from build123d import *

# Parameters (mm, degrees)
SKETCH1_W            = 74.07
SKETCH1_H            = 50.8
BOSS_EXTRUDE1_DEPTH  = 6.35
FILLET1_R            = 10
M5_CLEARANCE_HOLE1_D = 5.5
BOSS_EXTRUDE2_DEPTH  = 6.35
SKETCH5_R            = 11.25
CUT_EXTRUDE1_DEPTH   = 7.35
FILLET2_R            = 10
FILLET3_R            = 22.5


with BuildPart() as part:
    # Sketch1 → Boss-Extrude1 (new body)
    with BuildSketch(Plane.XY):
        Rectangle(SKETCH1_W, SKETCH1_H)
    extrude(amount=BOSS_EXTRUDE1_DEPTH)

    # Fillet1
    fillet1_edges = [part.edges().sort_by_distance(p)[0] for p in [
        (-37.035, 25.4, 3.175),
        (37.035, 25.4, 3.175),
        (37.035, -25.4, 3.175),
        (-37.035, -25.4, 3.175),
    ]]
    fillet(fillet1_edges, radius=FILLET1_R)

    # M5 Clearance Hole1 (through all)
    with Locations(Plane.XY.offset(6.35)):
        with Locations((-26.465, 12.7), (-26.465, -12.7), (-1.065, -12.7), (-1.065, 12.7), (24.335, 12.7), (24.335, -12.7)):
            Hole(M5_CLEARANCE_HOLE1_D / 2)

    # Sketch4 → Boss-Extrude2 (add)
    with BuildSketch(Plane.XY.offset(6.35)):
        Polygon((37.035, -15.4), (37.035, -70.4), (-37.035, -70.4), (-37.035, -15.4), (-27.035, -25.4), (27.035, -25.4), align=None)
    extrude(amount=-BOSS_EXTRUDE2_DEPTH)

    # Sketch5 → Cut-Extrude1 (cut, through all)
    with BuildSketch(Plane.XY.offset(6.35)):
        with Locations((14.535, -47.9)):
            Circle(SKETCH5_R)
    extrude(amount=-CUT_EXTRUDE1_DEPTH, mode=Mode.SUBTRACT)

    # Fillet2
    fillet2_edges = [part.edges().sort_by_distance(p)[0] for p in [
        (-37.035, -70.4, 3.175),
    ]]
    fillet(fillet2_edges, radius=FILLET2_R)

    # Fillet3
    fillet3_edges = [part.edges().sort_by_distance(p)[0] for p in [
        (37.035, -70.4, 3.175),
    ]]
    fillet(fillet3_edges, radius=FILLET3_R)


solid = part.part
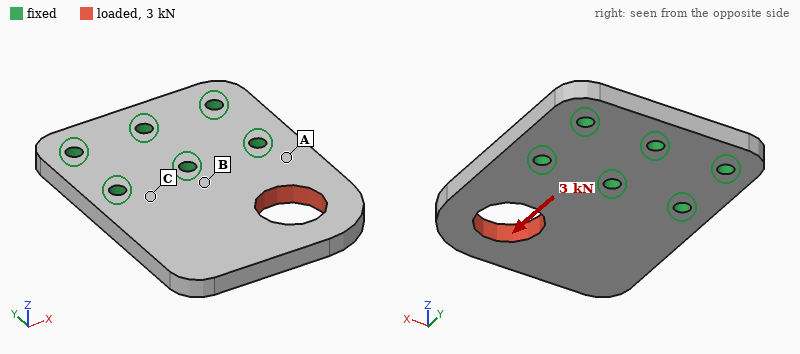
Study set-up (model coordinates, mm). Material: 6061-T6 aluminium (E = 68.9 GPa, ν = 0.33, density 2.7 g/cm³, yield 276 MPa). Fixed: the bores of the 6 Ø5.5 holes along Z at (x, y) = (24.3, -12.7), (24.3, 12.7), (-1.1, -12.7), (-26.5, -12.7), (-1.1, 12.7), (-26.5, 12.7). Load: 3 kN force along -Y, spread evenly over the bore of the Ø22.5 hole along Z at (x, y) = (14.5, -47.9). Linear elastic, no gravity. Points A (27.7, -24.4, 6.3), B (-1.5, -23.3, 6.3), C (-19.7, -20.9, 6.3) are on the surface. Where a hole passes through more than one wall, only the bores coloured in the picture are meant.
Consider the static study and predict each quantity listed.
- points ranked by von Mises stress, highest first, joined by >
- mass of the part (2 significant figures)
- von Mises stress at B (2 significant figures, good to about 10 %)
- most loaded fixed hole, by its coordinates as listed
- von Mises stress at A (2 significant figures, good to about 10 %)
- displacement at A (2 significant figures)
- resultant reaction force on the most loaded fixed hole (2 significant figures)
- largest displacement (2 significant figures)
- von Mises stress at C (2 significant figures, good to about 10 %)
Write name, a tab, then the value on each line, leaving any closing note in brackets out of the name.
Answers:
points ranked by von Mises stress, highest first, joined by >	A > B > C
mass of the part	110 g
von Mises stress at B	9.2 MPa
most loaded fixed hole, by its coordinates as listed	(24.3, -12.7)
von Mises stress at A	14 MPa
displacement at A	3.1 µm
resultant reaction force on the most loaded fixed hole	1.6 kN
largest displacement	13 µm
von Mises stress at C	3.3 MPa
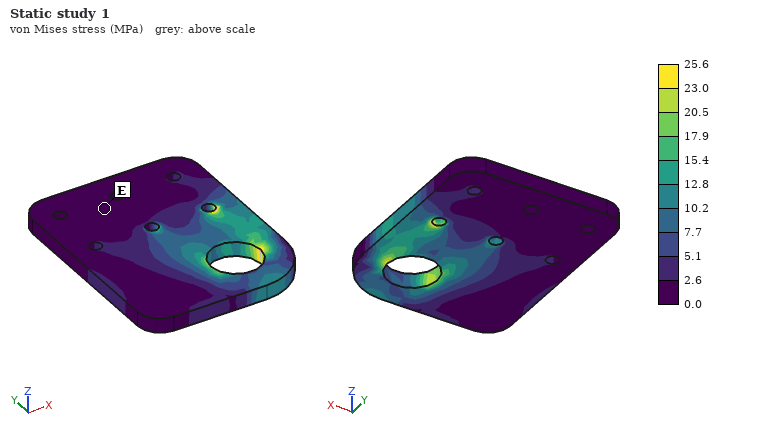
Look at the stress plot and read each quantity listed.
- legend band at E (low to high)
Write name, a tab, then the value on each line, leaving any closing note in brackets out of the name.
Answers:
legend band at E	0.0 to 2.6 MPa
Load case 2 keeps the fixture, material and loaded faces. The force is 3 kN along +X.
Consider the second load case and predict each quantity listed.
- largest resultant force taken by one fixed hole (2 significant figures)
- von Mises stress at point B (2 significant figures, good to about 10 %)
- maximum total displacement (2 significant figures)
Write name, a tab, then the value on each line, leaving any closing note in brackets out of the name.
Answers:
largest resultant force taken by one fixed hole	1.8 kN
von Mises stress at point B	14 MPa
maximum total displacement	26 µm
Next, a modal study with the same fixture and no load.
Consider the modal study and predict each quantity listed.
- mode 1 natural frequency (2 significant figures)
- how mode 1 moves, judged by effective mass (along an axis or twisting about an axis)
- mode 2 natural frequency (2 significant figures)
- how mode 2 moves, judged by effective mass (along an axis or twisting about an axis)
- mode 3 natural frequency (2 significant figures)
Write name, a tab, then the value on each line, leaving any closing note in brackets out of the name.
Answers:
mode 1 natural frequency	1700 Hz
how mode 1 moves, judged by effective mass	along Z
mode 2 natural frequency	3400 Hz
how mode 2 moves, judged by effective mass	twisting about Y
mode 3 natural frequency	7400 Hz
